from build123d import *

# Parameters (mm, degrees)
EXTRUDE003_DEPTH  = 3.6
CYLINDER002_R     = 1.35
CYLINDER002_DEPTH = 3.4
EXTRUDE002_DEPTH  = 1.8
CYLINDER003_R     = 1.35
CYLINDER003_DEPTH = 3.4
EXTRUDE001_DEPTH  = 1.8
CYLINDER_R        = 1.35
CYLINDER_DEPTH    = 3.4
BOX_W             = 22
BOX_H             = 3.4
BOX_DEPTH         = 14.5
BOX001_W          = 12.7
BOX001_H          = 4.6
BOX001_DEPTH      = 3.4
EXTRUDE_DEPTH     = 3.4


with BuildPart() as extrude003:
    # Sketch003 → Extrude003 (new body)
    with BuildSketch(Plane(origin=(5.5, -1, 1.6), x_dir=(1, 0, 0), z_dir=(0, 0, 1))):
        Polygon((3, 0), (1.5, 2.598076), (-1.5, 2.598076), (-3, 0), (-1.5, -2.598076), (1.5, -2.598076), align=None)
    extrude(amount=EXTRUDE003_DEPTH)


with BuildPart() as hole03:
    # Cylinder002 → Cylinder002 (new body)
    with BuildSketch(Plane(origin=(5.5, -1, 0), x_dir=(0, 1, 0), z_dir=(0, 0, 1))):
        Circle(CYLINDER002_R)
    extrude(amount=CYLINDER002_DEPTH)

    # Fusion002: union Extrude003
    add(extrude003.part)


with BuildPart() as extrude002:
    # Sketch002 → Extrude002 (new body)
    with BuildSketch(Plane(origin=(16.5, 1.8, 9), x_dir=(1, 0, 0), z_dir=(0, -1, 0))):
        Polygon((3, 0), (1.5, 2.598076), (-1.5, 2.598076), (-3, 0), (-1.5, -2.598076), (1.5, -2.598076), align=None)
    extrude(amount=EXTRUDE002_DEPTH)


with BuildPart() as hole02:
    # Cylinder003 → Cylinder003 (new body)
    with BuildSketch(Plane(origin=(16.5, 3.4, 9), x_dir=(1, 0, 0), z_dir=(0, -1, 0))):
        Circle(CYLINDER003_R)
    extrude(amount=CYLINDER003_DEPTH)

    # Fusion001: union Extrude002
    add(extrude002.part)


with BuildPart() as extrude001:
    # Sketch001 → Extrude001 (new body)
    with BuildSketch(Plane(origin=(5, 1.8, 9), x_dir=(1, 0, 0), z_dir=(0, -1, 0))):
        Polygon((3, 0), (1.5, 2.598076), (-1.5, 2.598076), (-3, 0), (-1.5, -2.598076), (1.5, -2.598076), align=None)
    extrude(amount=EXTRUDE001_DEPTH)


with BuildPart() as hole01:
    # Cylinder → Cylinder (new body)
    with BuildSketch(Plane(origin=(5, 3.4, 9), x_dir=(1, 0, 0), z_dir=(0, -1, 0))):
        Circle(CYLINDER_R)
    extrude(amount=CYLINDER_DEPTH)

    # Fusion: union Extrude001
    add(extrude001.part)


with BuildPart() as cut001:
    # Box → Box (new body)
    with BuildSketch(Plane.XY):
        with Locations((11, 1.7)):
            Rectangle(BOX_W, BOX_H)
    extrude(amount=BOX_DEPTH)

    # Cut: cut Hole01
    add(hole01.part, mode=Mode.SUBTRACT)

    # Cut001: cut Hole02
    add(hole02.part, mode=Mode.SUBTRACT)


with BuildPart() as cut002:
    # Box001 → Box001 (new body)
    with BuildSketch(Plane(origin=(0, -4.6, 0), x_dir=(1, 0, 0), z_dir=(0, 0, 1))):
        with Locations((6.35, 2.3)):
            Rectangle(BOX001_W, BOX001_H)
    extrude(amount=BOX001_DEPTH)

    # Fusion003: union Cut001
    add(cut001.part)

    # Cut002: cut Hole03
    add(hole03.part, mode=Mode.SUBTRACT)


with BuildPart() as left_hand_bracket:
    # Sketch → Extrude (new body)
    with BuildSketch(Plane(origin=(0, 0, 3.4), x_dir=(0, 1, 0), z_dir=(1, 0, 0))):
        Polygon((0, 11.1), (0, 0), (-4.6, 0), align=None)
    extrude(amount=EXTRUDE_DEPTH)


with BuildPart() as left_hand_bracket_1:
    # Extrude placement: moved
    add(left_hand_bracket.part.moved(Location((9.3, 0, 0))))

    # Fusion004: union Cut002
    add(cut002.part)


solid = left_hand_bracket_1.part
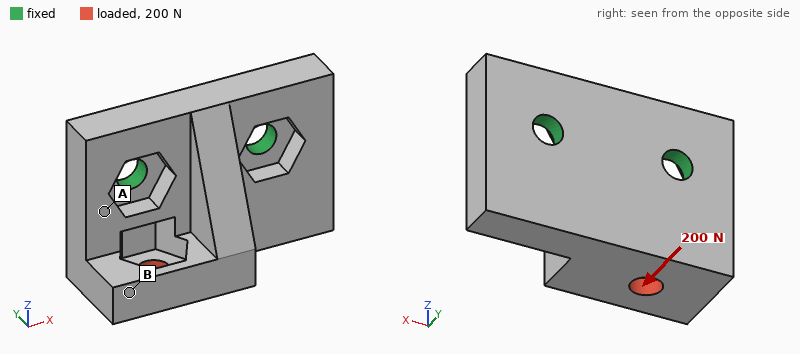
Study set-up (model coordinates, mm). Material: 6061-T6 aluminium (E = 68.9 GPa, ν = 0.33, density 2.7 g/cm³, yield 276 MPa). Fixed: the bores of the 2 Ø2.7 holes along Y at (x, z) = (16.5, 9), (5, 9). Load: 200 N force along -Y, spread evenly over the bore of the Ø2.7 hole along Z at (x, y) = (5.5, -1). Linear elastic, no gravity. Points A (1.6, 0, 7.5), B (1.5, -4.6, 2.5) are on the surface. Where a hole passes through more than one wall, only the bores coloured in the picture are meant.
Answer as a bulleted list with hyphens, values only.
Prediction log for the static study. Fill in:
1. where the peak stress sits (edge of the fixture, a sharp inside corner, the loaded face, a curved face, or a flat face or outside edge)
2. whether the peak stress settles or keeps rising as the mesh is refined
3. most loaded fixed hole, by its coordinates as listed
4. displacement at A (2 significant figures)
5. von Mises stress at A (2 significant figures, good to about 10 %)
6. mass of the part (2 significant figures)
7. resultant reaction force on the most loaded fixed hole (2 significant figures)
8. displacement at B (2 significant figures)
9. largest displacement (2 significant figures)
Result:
- edge of the fixture
- keeps rising
- (5, 9)
- 8.4 µm
- 44 MPa
- 3.3 g
- 190 N
- 32 µm
- 39 µm
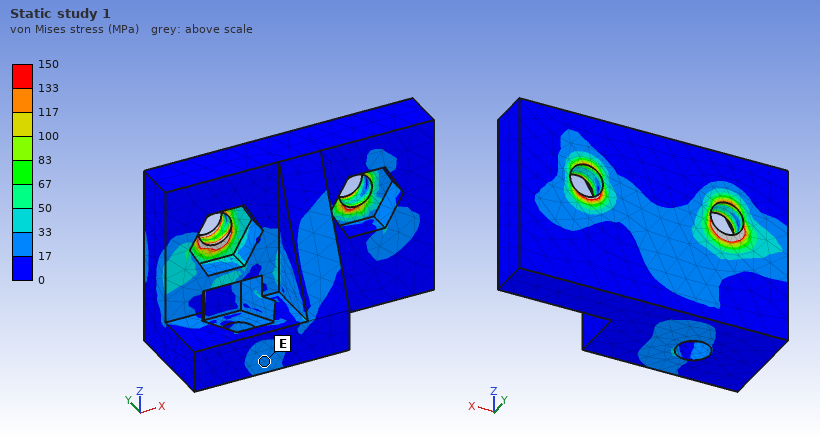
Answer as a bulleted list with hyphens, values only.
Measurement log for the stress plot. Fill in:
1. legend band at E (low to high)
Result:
- 17 to 33 MPa
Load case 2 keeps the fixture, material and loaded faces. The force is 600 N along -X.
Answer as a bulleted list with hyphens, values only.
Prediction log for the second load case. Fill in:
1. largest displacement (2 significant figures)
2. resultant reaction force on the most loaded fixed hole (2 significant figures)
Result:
- 19 µm
- 530 N
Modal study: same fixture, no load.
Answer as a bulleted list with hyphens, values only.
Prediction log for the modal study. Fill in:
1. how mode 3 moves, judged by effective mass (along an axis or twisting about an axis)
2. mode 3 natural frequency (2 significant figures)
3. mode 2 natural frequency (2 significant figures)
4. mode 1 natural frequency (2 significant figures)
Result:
- along X
- 38 kHz
- 25 kHz
- 13 kHz
